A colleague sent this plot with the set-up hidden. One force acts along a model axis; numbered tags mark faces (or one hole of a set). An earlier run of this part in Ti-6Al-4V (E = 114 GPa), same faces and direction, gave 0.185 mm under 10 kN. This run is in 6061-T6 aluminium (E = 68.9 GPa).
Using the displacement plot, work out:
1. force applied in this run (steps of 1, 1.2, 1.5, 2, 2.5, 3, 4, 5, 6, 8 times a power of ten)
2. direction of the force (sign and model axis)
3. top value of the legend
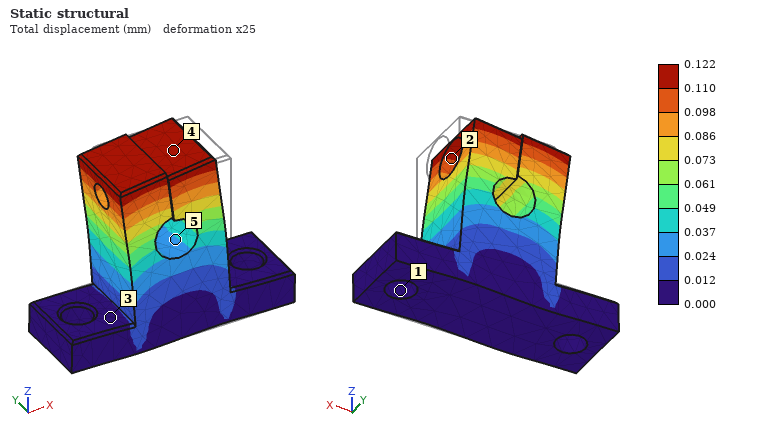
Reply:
4 kN
-X
0.122 mm
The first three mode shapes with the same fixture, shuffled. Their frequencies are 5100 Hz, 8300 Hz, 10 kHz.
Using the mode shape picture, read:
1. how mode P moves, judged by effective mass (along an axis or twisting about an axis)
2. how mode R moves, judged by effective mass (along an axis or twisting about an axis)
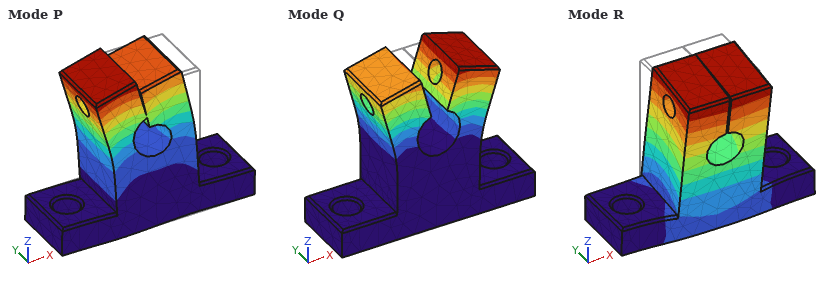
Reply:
along X
along Y
